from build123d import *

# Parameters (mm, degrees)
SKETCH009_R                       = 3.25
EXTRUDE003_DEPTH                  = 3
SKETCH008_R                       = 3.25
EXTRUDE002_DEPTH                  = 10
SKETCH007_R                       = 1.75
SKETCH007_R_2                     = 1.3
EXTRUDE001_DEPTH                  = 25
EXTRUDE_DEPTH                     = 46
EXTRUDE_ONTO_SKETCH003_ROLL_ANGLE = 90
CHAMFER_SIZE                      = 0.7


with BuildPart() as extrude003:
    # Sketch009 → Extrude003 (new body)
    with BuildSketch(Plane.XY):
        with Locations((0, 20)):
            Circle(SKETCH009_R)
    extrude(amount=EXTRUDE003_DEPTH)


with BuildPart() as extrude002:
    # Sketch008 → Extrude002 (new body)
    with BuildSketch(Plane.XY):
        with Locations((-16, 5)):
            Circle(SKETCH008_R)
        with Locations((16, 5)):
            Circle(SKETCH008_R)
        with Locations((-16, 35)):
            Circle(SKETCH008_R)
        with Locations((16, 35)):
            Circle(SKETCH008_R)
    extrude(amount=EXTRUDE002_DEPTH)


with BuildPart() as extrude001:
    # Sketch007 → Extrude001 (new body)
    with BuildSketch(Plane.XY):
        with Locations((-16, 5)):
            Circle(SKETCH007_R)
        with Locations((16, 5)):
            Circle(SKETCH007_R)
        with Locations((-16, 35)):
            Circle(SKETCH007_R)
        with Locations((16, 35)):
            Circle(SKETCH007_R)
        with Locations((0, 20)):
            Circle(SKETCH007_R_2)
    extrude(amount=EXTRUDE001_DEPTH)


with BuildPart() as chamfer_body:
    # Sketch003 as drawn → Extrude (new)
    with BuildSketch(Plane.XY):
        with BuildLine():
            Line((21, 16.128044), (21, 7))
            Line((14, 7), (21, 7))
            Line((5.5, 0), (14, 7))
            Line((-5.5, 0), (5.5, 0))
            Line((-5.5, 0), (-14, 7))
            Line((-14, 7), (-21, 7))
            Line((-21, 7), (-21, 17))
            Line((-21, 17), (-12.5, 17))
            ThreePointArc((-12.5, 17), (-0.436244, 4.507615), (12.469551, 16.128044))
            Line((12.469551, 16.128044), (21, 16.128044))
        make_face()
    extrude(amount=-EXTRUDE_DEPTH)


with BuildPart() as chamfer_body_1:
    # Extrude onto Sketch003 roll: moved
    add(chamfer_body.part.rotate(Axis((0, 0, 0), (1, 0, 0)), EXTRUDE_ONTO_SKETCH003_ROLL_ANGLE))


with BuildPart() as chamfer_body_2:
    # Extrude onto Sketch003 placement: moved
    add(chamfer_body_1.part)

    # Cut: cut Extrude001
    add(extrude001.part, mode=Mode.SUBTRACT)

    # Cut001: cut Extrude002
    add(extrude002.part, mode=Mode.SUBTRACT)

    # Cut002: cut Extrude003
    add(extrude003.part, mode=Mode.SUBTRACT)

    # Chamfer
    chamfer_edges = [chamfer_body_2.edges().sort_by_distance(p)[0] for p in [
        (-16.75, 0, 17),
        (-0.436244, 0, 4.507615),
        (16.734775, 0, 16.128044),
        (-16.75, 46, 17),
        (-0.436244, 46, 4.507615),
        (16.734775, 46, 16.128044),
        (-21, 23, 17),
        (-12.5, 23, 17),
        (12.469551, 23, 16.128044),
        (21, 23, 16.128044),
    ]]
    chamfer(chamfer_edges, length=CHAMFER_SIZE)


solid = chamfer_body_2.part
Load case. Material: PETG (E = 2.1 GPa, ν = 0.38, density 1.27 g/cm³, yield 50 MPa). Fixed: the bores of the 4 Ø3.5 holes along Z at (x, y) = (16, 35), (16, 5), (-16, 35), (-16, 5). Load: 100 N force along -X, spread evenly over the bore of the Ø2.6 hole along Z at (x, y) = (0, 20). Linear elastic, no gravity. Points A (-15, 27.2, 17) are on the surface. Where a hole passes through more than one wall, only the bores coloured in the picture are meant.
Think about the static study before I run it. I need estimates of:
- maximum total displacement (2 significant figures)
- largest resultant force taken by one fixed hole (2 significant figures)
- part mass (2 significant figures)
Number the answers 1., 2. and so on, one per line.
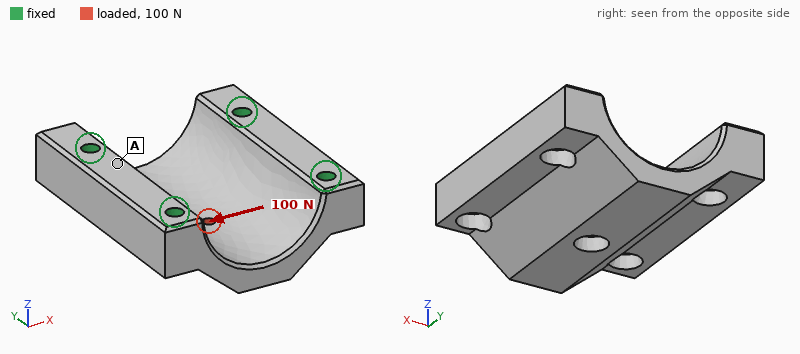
1. 23 µm
2. 29 N
3. 17 g
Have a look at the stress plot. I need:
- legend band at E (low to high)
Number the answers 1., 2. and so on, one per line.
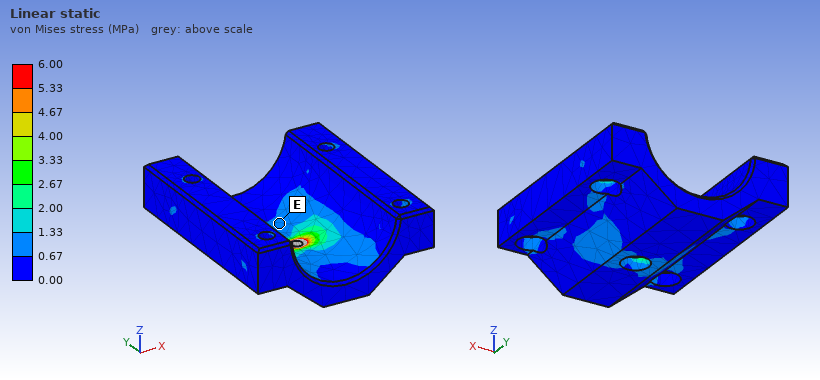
1. 0.67 to 1.33 MPa
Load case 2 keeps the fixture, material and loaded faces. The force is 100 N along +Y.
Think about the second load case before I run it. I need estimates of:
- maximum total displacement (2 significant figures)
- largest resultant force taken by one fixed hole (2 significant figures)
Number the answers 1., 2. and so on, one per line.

1. 20 µm
2. 32 N
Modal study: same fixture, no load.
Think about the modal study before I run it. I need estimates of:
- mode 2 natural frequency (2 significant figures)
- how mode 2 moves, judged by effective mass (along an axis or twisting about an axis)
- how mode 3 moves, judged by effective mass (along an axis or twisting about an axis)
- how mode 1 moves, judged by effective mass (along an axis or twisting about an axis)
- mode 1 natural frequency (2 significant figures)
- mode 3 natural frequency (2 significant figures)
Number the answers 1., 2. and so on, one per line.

1. 6500 Hz
2. along Y
3. along Z
4. along X
5. 6100 Hz
6. 7100 Hz
